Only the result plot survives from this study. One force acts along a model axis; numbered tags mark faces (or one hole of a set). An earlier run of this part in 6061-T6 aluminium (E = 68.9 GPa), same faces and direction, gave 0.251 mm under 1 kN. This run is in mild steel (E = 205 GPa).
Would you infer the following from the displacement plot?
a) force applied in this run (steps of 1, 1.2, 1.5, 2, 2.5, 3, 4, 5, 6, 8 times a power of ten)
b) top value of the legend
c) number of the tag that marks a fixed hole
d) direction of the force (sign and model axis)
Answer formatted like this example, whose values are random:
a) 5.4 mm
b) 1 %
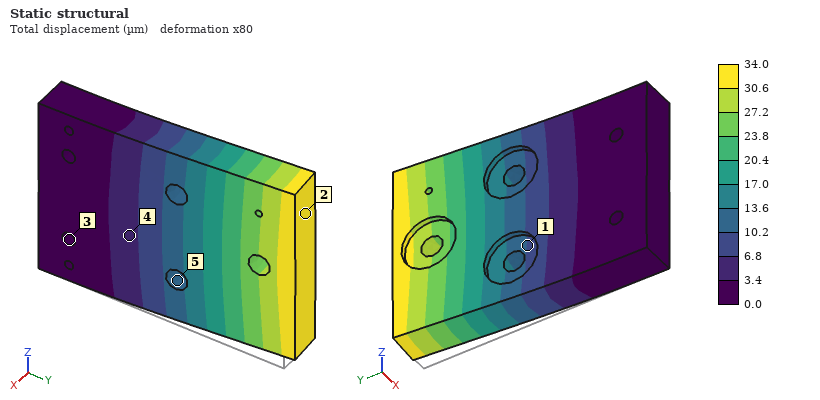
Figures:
a) 400 N
b) 34.0 µm
c) 3
d) -X
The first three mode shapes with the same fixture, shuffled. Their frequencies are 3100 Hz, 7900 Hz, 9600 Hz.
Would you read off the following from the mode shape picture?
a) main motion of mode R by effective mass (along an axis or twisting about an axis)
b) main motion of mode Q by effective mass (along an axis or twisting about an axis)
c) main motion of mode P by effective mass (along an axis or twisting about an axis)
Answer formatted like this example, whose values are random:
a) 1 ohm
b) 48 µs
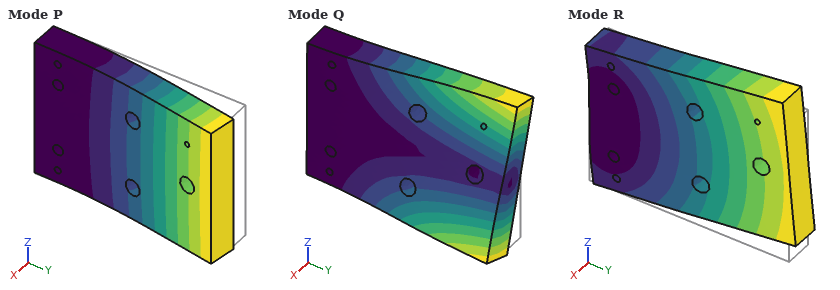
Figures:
a) along Z
b) twisting about Y
c) along X
